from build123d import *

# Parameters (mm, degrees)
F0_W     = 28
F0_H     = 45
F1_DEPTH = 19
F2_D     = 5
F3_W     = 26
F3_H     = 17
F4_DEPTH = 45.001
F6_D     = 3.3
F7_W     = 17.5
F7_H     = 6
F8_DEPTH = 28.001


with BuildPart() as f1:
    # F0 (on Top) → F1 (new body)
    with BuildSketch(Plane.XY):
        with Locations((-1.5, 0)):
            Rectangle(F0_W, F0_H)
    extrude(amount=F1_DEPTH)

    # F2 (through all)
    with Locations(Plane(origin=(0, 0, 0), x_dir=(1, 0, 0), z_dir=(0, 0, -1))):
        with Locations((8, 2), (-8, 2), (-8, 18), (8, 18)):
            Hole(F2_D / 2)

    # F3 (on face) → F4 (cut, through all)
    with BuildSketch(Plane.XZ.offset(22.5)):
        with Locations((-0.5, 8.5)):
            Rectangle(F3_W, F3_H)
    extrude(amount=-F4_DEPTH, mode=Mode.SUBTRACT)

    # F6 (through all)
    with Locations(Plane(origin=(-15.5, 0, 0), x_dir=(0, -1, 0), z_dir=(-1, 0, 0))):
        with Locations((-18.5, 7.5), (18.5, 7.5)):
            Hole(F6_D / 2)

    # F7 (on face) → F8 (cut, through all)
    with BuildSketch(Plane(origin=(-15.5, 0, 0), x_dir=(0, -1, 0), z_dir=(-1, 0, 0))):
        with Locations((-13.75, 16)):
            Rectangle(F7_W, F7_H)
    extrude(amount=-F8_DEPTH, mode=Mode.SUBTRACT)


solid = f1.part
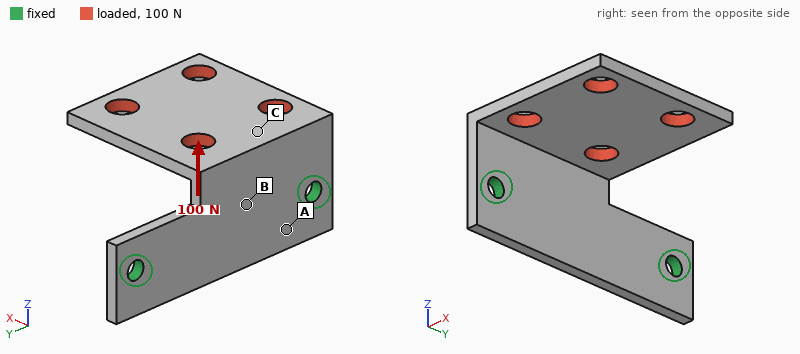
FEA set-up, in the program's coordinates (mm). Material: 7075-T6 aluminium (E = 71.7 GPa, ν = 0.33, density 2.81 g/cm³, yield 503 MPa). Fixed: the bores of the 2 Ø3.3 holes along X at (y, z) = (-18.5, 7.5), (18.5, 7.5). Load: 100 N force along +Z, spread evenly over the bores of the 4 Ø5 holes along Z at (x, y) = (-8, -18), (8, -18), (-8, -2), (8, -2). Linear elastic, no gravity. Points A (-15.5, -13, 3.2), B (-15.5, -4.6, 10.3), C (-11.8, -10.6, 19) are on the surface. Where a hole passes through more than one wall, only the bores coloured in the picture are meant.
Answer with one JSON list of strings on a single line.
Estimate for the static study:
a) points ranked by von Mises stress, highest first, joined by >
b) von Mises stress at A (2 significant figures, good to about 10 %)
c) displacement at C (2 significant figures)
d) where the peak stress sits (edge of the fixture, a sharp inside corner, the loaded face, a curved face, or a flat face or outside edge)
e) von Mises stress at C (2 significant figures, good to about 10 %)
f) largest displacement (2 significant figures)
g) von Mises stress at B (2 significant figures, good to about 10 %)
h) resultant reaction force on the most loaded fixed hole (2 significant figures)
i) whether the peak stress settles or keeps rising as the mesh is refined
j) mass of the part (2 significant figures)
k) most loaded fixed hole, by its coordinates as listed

["C > B > A", "22 MPa", "0.100 mm", "edge of the fixture", "73 MPa", "0.58 mm", "43 MPa", "78 N", "keeps rising", "7.7 g", "(-18.5, 7.5)"]
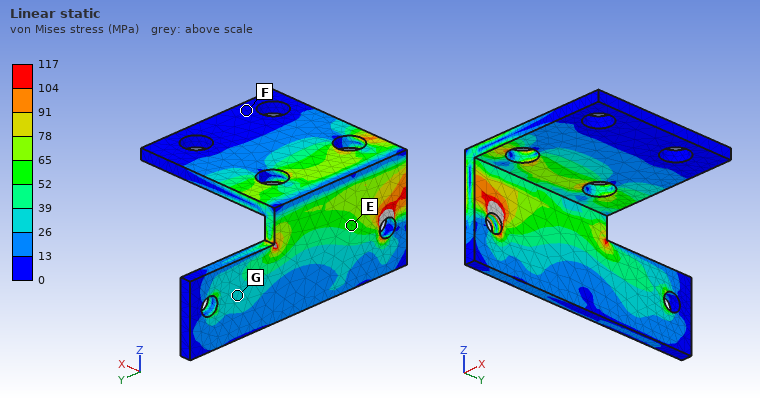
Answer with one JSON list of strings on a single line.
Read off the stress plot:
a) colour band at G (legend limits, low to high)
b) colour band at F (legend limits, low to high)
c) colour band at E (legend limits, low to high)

["26 to 39 MPa", "0 to 13 MPa", "52 to 65 MPa"]
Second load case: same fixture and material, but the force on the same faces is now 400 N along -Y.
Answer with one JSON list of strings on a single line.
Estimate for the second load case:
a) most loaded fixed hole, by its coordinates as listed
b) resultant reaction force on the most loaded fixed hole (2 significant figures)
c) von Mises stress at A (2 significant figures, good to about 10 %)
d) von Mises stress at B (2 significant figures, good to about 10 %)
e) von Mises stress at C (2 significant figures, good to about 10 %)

["(-18.5, 7.5)", "340 N", "53 MPa", "75 MPa", "62 MPa"]
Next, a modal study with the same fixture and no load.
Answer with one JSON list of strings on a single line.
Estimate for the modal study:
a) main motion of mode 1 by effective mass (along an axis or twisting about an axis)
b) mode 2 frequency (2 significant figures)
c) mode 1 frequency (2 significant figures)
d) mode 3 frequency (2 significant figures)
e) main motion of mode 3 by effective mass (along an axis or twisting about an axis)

["along Z", "2700 Hz", "1400 Hz", "4600 Hz", "along X"]
